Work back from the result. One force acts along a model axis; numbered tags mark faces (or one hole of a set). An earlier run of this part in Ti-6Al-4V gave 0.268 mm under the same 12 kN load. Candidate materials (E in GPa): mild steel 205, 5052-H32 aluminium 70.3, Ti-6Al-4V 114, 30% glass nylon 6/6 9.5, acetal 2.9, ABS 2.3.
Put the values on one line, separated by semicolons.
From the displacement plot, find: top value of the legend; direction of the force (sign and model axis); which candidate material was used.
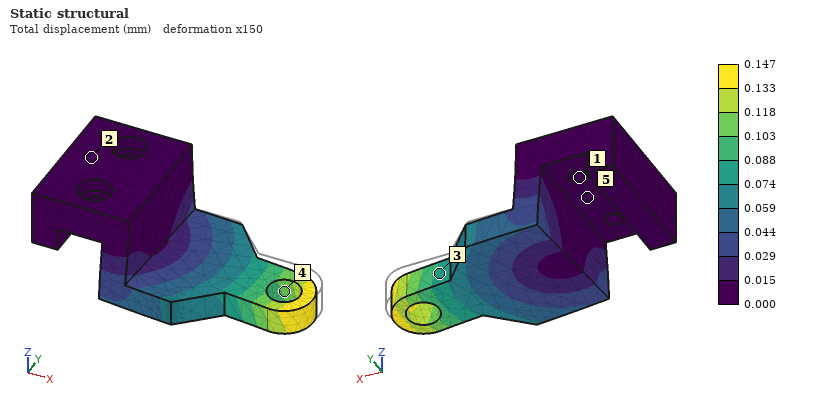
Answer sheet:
0.147 mm; -Y; mild steel
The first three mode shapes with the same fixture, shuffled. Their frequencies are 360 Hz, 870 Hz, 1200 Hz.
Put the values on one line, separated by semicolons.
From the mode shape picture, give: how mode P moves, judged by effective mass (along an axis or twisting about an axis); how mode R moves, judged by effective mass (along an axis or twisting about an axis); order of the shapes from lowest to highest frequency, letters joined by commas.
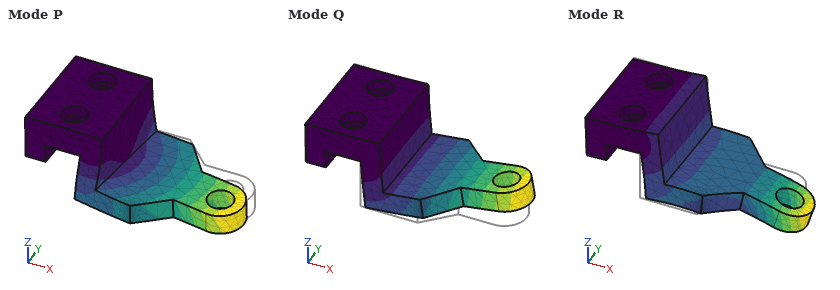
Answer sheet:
along Y; along X; Q, P, R
